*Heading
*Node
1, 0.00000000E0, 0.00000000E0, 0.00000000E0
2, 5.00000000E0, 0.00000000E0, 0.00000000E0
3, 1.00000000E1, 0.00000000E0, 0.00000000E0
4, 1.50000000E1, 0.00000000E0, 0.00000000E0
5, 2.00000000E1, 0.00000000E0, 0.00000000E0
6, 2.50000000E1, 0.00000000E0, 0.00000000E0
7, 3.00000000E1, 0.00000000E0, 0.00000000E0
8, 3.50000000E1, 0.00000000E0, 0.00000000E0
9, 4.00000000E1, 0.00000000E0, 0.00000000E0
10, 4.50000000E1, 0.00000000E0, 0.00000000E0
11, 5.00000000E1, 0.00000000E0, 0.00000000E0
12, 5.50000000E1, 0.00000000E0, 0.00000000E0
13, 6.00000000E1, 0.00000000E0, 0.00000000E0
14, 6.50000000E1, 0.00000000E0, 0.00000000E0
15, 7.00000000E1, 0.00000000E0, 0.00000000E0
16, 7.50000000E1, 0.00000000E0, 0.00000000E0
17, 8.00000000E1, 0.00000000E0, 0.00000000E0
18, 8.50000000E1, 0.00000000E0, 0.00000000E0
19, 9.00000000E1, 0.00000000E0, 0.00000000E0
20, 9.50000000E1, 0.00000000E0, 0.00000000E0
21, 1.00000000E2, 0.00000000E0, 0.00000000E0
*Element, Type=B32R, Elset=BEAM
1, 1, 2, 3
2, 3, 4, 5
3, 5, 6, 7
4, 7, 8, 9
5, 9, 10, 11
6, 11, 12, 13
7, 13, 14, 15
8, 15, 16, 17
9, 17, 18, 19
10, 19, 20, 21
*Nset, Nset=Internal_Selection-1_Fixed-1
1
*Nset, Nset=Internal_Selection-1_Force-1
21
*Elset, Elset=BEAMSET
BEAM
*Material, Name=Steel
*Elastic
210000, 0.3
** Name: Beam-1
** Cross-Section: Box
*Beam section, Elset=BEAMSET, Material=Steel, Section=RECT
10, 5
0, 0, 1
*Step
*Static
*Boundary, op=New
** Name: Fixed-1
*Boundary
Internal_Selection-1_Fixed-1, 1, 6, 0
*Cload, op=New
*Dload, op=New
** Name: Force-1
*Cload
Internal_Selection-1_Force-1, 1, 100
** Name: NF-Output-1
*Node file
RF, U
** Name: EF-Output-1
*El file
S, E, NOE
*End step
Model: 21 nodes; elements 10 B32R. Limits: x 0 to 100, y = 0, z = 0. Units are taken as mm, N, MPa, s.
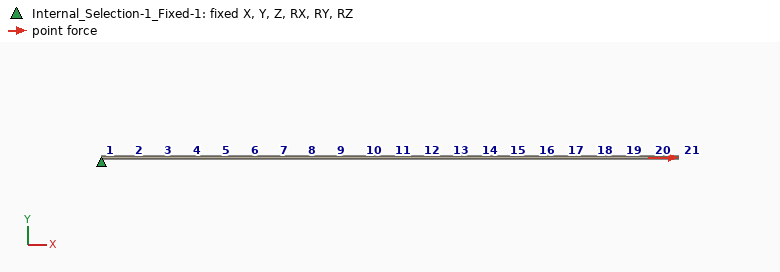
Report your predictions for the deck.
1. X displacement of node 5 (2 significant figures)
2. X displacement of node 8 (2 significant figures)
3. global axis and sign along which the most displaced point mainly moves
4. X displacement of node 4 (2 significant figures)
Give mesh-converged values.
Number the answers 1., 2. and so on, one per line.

1. 1.9e-04 mm
2. 3.3e-04 mm
3. +X
4. 1.4e-04 mm
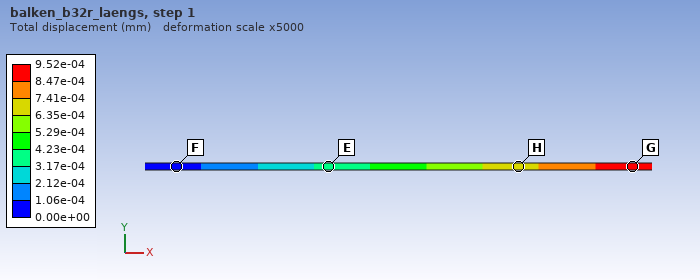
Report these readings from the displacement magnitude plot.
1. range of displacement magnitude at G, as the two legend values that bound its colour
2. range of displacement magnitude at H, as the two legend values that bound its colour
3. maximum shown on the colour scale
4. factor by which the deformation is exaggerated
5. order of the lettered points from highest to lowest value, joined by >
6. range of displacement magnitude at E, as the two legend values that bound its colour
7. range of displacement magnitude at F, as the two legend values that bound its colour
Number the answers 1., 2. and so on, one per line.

1. 8.47e-04 to 9.52e-04 mm
2. 6.35e-04 to 7.41e-04 mm
3. 9.52e-04 mm
4. 5000
5. G > H > E > F
6. 3.17e-04 to 4.23e-04 mm
7. 0.00e+00 to 1.06e-04 mm
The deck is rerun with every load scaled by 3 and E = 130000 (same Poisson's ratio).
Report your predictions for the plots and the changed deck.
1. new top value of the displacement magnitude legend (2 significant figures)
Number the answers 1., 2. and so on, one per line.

1. 0.0046 mm
